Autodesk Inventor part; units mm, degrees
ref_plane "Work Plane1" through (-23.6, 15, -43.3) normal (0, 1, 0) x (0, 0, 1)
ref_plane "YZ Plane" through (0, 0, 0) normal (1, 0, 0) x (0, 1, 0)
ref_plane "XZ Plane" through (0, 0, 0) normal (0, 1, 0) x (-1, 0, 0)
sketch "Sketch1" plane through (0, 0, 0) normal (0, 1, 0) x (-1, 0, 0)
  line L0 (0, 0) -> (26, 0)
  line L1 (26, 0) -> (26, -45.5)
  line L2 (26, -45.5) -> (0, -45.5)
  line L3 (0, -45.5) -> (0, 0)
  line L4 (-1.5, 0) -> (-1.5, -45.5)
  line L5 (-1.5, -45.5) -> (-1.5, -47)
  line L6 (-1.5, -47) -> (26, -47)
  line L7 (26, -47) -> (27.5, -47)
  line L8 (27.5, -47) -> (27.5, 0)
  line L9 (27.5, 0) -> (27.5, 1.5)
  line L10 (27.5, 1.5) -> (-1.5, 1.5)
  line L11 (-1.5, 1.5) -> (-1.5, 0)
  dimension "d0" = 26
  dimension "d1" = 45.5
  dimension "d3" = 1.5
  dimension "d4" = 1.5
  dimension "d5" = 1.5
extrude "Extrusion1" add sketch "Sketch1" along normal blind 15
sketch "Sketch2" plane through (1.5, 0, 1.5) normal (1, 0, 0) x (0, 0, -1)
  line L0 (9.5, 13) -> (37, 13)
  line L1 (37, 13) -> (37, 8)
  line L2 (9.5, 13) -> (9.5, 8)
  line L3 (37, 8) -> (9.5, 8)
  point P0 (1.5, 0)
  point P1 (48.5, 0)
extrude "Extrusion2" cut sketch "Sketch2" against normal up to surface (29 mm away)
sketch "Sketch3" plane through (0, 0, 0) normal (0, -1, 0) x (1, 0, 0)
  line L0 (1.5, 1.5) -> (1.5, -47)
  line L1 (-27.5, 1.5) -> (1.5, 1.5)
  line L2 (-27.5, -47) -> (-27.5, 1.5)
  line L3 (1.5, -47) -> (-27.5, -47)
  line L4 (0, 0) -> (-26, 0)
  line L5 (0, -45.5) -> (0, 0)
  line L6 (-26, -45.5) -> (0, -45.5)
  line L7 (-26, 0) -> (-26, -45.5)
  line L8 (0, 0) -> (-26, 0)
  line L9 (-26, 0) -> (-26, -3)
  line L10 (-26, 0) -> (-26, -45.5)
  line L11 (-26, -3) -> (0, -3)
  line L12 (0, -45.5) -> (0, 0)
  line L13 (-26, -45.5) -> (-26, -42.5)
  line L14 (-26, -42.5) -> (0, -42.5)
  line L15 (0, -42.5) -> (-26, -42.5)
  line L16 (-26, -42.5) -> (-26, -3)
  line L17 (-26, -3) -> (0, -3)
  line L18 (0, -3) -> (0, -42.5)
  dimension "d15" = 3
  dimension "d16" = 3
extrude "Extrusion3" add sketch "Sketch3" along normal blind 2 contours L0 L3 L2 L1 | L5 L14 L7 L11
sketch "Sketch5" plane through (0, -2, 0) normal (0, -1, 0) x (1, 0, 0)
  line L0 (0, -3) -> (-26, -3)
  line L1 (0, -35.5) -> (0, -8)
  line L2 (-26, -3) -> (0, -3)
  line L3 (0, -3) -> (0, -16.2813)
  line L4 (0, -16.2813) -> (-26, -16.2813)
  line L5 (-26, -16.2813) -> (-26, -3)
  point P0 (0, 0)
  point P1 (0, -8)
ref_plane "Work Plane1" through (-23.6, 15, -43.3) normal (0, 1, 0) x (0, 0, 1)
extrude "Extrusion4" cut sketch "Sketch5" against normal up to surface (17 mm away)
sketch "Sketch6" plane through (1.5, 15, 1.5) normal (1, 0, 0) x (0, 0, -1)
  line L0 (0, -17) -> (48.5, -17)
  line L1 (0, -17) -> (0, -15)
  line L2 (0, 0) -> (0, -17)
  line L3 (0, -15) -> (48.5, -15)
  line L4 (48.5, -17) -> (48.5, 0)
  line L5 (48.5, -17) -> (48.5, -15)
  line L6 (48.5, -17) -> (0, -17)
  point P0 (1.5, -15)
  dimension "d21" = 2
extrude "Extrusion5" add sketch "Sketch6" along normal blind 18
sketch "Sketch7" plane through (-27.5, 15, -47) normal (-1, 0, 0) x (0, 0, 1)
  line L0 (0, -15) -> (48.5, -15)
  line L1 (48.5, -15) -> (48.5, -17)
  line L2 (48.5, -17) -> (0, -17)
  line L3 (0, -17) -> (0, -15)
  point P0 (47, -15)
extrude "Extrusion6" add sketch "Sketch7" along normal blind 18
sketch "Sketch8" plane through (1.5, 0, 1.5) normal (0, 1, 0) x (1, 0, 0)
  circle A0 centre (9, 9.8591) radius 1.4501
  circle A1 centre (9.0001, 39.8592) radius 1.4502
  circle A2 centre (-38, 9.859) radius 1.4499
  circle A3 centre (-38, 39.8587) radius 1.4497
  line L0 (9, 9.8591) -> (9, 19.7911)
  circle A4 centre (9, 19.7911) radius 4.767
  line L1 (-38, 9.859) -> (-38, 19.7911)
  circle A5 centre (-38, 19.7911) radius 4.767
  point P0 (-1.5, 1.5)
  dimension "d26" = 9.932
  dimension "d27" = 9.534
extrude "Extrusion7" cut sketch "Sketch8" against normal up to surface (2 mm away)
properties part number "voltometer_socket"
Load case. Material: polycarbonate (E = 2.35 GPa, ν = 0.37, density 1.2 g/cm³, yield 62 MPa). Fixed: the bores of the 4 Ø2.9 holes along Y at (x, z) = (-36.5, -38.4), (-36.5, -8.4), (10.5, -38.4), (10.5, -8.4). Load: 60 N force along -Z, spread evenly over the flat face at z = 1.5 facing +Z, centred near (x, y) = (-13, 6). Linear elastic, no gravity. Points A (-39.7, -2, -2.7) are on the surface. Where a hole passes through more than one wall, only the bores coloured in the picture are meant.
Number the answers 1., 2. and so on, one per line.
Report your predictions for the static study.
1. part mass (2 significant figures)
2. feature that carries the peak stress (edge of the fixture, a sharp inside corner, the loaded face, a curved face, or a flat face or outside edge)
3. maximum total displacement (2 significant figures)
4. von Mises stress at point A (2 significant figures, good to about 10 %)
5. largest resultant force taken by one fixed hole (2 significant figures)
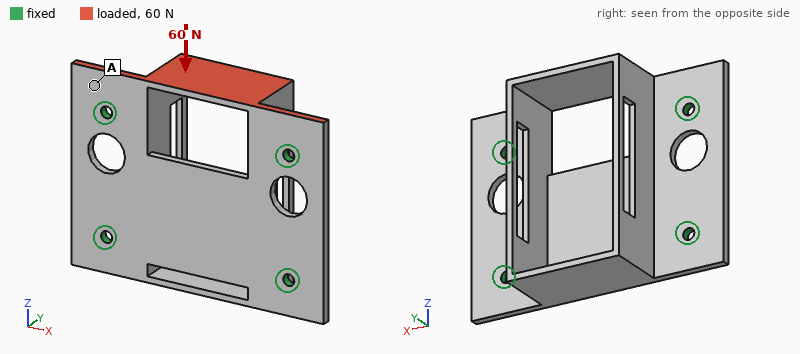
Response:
1. 9.5 g
2. the loaded face
3. 0.56 mm
4. 1.6 MPa
5. 17 N
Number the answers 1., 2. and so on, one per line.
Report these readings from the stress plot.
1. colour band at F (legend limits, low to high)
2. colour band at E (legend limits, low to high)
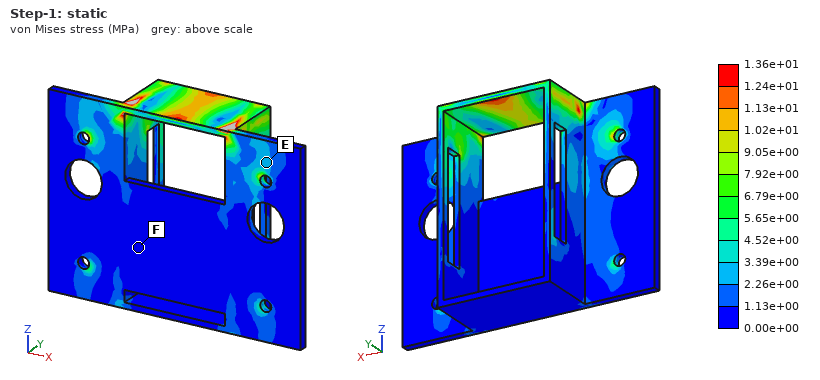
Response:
1. 0.00e+00 to 1.13e+00 MPa
2. 2.26e+00 to 3.39e+00 MPa
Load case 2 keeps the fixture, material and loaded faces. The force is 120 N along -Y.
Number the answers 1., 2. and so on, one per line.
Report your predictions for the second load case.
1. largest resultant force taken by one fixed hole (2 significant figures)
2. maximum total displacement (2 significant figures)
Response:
1. 84 N
2. 0.84 mm
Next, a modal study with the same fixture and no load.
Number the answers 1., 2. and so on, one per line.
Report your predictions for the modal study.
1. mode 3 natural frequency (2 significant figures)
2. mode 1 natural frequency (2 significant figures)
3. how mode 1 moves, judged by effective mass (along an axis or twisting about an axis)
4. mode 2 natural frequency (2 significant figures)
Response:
1. 1600 Hz
2. 1200 Hz
3. along Y
4. 1400 Hz
